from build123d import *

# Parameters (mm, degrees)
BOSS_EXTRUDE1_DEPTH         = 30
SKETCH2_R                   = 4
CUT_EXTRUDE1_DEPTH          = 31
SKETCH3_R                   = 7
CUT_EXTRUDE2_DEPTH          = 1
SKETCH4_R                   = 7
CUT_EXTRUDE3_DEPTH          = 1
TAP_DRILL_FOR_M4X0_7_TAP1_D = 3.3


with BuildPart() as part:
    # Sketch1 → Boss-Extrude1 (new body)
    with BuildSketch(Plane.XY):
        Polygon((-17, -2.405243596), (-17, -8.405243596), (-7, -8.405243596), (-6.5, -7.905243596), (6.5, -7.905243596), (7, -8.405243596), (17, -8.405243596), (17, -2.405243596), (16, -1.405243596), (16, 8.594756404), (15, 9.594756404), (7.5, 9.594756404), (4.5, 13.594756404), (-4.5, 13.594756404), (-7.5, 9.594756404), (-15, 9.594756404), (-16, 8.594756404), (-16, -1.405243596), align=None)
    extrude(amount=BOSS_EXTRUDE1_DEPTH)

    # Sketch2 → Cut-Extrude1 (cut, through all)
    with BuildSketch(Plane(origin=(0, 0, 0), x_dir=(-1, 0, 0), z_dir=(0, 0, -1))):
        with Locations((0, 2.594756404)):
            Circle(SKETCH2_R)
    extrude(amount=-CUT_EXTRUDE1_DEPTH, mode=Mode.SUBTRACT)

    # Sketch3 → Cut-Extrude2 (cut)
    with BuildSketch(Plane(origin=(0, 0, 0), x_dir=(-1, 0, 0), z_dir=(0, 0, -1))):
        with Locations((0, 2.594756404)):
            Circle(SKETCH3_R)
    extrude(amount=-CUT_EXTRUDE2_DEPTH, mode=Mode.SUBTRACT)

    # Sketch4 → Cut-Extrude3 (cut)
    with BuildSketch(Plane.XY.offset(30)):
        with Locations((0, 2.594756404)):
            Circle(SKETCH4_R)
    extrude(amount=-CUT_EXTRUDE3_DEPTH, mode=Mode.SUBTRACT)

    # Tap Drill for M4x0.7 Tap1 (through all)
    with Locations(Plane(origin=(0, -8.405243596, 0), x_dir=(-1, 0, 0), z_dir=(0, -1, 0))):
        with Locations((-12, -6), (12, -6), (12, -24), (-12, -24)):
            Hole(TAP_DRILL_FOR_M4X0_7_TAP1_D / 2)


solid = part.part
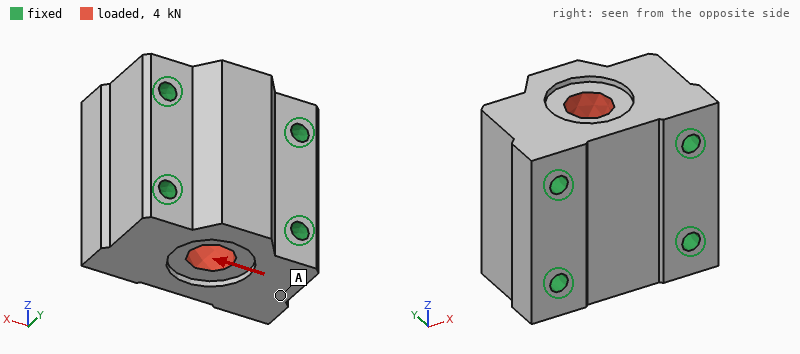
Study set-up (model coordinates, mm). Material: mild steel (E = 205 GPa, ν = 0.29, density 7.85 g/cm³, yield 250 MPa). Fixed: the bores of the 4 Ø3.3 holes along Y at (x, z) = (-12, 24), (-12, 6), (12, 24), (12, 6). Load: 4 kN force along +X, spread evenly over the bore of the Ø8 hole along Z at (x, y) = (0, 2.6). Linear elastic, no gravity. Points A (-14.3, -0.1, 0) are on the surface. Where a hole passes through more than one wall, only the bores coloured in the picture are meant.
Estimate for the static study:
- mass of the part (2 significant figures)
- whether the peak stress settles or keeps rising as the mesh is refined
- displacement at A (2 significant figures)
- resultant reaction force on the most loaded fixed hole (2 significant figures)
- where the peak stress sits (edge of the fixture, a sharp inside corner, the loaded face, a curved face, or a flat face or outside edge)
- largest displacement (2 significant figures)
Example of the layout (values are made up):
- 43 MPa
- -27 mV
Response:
- 130 g
- keeps rising
- 0.078 µm
- 1.0 kN
- edge of the fixture
- 0.40 µm
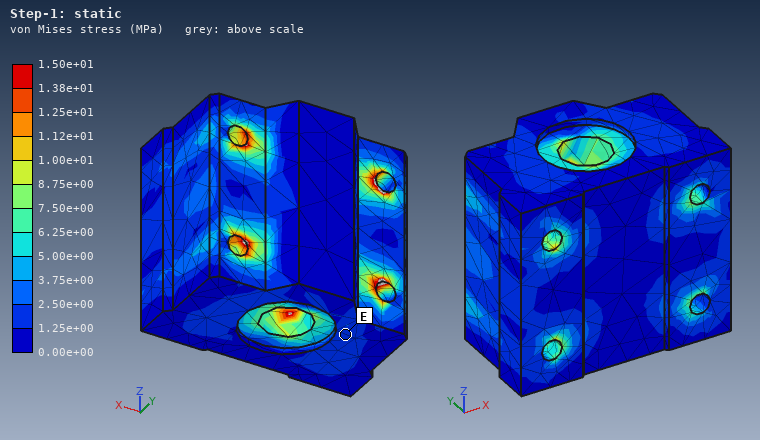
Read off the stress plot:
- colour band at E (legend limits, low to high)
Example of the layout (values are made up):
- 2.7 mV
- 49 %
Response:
- 1.25e+00 to 2.50e+00 MPa
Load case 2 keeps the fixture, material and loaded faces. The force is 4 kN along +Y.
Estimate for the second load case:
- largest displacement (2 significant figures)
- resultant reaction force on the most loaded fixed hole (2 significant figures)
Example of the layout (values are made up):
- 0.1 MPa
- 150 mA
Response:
- 0.72 µm
- 1.0 kN
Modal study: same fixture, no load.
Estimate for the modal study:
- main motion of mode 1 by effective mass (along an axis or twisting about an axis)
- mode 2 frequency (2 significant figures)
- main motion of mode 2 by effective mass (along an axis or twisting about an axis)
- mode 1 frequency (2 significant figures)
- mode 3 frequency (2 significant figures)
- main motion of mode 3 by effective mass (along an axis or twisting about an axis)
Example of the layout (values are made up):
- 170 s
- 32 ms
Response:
- along Z
- 55 kHz
- along Y
- 51 kHz
- 63 kHz
- along Z
